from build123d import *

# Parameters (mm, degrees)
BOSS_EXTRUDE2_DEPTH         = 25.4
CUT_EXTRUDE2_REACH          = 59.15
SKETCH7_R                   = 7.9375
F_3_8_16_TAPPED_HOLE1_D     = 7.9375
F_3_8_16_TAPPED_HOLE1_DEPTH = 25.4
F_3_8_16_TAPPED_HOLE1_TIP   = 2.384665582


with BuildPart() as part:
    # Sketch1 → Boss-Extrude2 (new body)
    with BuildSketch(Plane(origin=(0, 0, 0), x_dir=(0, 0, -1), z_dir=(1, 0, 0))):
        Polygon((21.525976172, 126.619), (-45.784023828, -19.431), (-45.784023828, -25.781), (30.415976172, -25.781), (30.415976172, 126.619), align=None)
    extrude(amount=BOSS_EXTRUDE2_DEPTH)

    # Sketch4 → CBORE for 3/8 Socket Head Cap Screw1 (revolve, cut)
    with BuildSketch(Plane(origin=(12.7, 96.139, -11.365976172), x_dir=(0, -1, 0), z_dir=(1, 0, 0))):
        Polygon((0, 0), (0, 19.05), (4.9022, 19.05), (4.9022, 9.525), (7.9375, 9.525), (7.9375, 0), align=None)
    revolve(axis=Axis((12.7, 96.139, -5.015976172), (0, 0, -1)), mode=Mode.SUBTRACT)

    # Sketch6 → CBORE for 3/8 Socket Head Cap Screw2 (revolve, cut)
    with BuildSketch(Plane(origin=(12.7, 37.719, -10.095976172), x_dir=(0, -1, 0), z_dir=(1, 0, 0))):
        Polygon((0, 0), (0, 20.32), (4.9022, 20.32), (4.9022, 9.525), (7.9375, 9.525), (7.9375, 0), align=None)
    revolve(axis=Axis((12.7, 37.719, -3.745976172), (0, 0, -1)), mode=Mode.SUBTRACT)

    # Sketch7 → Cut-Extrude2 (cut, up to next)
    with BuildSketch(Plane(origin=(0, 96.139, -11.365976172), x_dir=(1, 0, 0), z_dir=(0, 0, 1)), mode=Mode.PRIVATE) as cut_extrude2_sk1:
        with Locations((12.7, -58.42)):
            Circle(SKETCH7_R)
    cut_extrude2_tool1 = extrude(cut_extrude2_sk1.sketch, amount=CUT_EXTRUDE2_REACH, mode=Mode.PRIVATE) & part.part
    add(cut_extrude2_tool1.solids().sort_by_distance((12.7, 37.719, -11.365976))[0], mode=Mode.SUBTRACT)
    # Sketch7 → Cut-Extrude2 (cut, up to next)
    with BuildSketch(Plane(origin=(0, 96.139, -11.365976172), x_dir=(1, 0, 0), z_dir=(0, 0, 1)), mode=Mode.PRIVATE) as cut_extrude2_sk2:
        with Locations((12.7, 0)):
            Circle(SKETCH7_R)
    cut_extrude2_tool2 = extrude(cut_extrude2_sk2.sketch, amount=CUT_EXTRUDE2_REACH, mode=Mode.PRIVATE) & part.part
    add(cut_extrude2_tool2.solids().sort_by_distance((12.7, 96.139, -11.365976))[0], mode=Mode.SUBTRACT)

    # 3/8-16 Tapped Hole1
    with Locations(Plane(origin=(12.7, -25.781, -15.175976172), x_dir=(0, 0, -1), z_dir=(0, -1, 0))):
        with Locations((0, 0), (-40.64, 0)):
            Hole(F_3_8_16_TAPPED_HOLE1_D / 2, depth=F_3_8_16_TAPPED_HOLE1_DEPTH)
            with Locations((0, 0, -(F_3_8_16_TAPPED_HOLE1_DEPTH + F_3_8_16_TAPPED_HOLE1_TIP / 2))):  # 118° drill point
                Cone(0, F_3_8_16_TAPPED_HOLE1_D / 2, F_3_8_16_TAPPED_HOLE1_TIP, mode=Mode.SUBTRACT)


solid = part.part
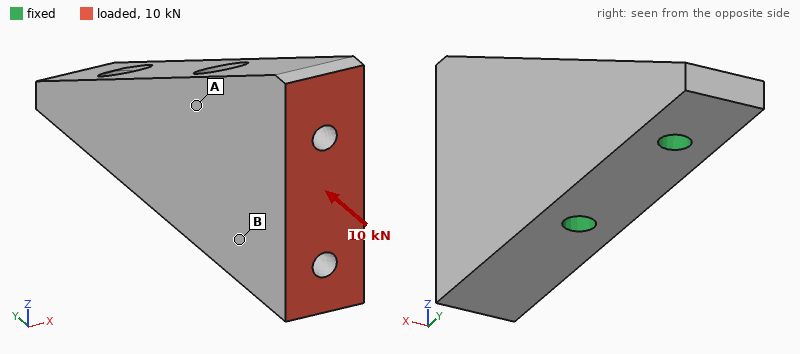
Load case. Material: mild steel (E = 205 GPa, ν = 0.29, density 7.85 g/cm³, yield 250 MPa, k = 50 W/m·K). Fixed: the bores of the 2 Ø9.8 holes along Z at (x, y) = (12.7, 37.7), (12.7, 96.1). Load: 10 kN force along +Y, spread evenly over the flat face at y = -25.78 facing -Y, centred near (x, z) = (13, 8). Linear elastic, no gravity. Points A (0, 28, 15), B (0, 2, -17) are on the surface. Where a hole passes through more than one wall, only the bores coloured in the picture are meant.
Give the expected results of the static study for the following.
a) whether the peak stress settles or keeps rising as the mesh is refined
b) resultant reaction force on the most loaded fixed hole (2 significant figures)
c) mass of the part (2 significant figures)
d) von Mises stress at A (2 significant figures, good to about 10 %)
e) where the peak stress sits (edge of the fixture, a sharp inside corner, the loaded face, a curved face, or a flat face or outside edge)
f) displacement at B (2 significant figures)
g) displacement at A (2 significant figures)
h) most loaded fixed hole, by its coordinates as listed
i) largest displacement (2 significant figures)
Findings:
keeps rising
7.6 kN
1.2 kg
34 MPa
edge of the fixture
12 µm
13 µm
(12.7, 96.1)
35 µm
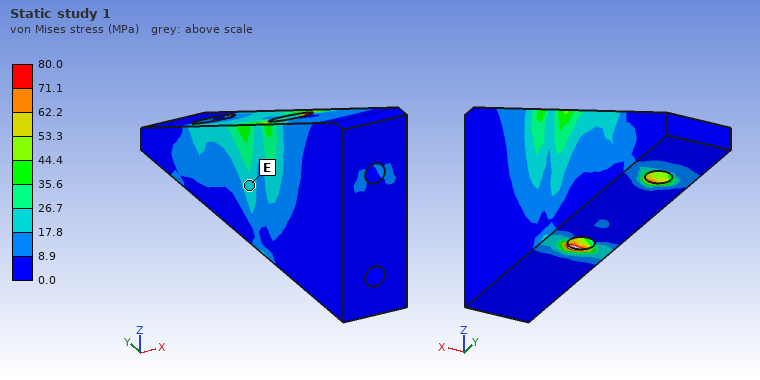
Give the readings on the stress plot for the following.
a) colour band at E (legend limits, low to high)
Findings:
17.8 to 26.7 MPa
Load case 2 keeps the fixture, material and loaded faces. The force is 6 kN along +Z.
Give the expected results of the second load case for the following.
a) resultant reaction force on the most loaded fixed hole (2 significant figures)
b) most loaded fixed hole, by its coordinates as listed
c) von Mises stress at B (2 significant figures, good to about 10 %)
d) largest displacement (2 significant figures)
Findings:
13 kN
(12.7, 37.7)
13 MPa
51 µm
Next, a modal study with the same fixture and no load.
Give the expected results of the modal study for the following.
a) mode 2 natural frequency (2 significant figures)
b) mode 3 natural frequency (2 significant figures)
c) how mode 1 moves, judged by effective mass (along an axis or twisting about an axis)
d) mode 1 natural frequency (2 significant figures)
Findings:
3100 Hz
4300 Hz
along X
1900 Hz
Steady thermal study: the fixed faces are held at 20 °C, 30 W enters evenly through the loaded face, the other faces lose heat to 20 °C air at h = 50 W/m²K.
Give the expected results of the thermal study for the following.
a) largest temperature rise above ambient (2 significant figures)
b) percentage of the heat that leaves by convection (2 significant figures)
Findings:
29 K
44 %
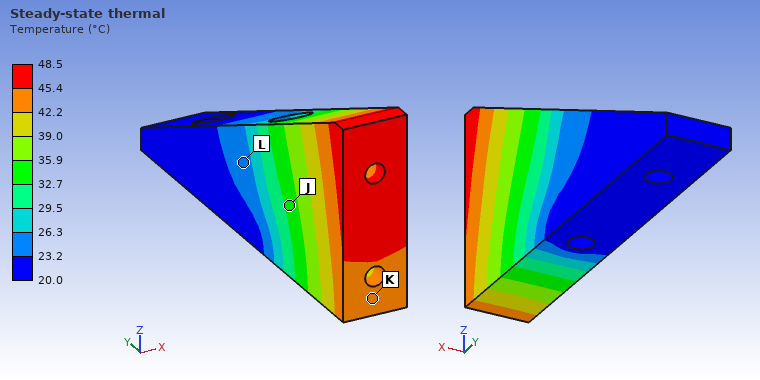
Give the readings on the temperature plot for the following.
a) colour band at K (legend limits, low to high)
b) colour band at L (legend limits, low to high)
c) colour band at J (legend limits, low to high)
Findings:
42.2 to 45.4 °C
23.2 to 26.3 °C
32.7 to 35.9 °C
